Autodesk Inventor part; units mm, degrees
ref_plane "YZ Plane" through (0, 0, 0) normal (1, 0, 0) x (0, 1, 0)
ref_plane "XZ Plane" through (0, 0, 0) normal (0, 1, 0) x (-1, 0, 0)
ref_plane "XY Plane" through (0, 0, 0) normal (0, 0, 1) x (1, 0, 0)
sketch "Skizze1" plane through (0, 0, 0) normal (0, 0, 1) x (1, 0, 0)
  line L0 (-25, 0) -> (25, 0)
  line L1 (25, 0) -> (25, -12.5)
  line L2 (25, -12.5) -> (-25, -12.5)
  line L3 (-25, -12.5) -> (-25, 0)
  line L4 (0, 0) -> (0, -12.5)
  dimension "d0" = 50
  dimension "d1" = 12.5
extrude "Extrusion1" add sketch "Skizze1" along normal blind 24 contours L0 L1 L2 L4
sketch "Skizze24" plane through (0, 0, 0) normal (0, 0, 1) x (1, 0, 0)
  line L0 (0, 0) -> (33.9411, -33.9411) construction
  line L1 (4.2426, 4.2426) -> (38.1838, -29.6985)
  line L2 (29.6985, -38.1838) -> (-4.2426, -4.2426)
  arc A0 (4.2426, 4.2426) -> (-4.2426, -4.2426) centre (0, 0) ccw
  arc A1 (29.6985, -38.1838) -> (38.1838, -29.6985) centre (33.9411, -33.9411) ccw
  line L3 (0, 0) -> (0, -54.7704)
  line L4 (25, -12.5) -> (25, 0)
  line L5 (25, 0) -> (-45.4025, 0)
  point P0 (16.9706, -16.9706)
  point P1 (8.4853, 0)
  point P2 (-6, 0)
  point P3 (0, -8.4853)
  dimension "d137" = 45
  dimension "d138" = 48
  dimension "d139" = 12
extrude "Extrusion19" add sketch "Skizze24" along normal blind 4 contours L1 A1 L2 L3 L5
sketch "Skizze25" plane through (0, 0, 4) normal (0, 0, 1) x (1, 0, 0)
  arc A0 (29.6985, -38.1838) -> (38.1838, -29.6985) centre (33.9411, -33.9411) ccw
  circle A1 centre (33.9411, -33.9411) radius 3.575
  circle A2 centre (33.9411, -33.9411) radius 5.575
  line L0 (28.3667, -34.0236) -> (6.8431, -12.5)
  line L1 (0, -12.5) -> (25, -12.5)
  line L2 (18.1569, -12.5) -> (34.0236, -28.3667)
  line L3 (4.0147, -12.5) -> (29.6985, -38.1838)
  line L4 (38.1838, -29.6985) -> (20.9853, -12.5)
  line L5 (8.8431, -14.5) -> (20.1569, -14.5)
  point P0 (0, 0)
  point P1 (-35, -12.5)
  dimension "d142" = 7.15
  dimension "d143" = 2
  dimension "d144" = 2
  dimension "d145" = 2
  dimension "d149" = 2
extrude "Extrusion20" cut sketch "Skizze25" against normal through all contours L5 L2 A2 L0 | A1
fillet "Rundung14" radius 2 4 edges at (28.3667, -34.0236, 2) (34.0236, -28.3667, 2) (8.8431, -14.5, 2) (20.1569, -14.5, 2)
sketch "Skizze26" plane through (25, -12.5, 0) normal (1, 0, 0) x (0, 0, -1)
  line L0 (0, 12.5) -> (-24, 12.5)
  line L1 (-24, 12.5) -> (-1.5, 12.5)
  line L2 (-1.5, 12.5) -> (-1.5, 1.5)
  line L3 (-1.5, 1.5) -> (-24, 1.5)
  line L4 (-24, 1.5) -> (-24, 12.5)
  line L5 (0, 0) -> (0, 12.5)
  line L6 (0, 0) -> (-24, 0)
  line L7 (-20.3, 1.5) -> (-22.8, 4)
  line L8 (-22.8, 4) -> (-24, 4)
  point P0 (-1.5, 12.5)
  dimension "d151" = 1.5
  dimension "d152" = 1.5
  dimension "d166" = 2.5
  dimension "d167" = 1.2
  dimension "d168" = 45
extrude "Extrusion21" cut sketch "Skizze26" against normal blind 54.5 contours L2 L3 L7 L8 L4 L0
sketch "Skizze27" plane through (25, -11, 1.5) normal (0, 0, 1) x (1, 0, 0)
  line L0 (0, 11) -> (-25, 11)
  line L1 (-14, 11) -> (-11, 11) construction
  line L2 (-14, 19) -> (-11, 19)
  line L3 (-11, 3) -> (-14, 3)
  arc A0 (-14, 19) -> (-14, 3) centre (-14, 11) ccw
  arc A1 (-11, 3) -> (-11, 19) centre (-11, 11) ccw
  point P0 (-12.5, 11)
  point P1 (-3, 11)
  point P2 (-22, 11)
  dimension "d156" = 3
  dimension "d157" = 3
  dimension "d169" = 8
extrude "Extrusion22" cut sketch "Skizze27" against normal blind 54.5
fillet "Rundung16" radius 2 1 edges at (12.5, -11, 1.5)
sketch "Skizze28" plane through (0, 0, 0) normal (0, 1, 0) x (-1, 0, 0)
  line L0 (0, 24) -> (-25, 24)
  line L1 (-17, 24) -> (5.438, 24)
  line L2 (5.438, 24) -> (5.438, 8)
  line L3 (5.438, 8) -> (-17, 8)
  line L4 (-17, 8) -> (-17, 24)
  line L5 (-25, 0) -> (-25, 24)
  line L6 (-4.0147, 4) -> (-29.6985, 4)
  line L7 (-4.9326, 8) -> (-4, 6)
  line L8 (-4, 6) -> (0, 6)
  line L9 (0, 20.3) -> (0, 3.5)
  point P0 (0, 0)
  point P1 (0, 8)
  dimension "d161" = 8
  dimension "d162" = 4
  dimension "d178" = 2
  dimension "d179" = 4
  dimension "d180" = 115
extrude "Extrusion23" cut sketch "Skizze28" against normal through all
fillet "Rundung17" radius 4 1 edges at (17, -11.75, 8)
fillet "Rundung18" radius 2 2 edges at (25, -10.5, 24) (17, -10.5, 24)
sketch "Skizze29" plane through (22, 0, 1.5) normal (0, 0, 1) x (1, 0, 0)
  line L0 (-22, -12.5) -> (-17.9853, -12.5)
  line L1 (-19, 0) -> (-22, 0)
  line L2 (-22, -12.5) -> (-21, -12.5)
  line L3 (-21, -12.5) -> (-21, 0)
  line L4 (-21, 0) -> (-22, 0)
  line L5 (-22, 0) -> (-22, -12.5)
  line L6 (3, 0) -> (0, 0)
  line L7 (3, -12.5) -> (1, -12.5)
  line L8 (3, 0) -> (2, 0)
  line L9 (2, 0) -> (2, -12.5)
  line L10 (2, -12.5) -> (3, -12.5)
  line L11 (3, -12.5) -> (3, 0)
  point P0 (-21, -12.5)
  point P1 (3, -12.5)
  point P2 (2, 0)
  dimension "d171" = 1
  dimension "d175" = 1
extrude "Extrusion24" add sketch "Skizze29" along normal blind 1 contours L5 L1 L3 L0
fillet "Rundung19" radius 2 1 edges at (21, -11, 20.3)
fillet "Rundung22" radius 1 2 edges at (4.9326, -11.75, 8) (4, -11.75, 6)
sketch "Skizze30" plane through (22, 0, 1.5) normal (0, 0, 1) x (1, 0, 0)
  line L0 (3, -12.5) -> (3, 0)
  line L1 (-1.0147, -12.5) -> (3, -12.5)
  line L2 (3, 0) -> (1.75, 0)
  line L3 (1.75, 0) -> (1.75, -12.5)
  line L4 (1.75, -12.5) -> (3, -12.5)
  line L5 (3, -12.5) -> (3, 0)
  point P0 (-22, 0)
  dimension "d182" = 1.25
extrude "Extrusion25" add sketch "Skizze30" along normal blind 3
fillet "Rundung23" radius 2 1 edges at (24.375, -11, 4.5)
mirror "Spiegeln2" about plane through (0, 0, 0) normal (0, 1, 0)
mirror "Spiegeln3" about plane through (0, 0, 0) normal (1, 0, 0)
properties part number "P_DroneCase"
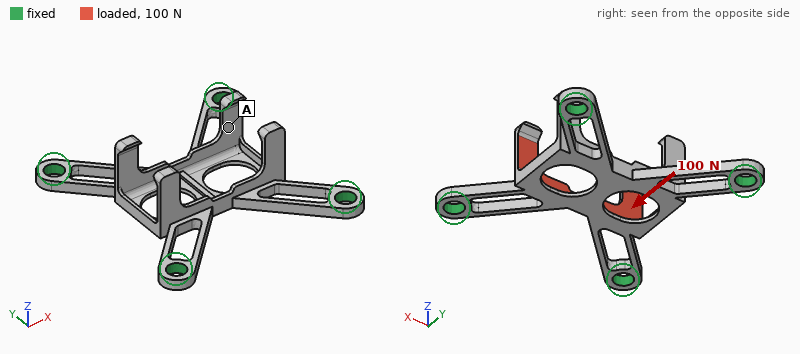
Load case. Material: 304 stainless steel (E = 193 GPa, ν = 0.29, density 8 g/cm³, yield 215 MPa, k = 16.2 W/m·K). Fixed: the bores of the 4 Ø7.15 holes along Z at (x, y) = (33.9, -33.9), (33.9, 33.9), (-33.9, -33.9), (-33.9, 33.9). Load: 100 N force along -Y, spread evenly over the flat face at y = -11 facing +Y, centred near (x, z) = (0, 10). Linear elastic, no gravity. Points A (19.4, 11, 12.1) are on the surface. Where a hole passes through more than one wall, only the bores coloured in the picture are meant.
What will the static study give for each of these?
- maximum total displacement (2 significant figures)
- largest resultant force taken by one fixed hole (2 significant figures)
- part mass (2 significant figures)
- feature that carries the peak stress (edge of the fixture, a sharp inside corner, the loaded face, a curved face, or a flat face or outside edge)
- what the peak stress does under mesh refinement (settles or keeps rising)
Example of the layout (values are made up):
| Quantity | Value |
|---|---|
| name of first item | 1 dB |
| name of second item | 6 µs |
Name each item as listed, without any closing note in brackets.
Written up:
| Quantity | Value |
|---|---|
| maximum total displacement | 56 µm |
| largest resultant force taken by one fixed hole | 66 N |
| part mass | 53 g |
| feature that carries the peak stress | a sharp inside corner |
| what the peak stress does under mesh refinement | keeps rising |
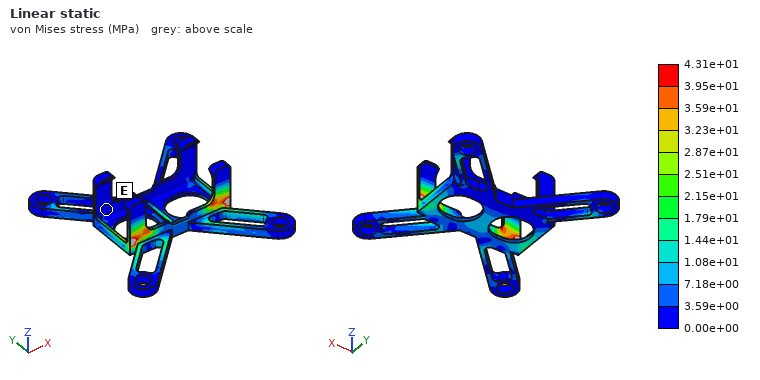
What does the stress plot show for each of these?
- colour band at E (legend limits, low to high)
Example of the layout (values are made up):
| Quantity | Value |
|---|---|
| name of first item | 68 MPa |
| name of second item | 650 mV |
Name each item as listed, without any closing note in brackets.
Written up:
| Quantity | Value |
|---|---|
| colour band at E | 0.00e+00 to 3.59e+00 MPa |
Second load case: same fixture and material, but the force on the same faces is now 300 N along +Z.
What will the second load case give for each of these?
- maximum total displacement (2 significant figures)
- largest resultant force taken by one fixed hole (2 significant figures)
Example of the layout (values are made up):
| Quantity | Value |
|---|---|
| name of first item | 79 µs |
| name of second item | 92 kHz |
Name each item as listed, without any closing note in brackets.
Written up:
| Quantity | Value |
|---|---|
| maximum total displacement | 88 µm |
| largest resultant force taken by one fixed hole | 150 N |
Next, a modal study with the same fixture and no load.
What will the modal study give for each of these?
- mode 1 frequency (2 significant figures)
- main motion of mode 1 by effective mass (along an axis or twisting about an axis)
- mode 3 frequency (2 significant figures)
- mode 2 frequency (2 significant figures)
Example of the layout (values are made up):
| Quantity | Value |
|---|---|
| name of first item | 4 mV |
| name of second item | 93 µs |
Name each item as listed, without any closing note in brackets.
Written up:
| Quantity | Value |
|---|---|
| mode 1 frequency | 1900 Hz |
| main motion of mode 1 by effective mass | along Z |
| mode 3 frequency | 2400 Hz |
| mode 2 frequency | 2200 Hz |
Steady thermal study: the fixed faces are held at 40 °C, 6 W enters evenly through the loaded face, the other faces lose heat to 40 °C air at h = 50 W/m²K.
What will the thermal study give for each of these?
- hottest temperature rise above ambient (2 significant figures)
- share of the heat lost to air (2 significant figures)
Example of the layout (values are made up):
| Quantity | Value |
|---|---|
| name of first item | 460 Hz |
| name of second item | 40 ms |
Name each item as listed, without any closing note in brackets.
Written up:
| Quantity | Value |
|---|---|
| hottest temperature rise above ambient | 66 K |
| share of the heat lost to air | 91 % |
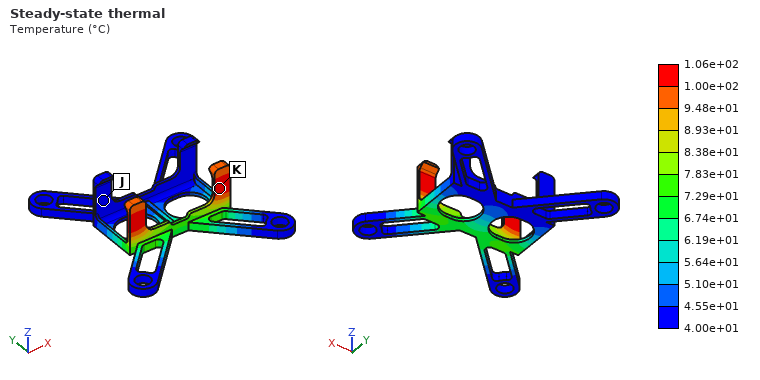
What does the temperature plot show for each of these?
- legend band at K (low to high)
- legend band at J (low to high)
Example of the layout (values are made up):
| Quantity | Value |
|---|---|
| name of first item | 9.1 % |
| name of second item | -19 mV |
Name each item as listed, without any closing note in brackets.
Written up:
| Quantity | Value |
|---|---|
| legend band at K | 1.00e+02 to 1.06e+02 °C |
| legend band at J | 4.00e+01 to 4.55e+01 °C |
